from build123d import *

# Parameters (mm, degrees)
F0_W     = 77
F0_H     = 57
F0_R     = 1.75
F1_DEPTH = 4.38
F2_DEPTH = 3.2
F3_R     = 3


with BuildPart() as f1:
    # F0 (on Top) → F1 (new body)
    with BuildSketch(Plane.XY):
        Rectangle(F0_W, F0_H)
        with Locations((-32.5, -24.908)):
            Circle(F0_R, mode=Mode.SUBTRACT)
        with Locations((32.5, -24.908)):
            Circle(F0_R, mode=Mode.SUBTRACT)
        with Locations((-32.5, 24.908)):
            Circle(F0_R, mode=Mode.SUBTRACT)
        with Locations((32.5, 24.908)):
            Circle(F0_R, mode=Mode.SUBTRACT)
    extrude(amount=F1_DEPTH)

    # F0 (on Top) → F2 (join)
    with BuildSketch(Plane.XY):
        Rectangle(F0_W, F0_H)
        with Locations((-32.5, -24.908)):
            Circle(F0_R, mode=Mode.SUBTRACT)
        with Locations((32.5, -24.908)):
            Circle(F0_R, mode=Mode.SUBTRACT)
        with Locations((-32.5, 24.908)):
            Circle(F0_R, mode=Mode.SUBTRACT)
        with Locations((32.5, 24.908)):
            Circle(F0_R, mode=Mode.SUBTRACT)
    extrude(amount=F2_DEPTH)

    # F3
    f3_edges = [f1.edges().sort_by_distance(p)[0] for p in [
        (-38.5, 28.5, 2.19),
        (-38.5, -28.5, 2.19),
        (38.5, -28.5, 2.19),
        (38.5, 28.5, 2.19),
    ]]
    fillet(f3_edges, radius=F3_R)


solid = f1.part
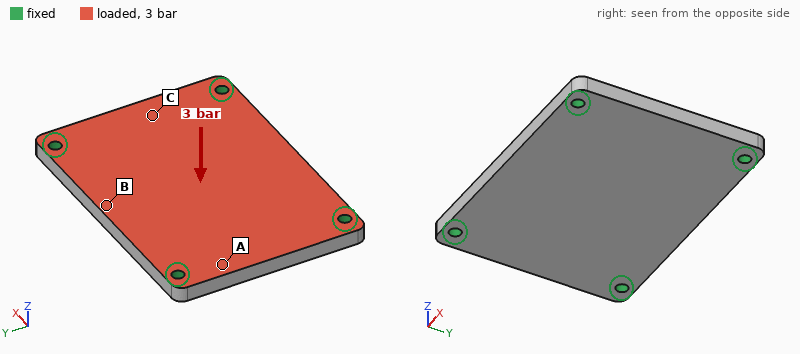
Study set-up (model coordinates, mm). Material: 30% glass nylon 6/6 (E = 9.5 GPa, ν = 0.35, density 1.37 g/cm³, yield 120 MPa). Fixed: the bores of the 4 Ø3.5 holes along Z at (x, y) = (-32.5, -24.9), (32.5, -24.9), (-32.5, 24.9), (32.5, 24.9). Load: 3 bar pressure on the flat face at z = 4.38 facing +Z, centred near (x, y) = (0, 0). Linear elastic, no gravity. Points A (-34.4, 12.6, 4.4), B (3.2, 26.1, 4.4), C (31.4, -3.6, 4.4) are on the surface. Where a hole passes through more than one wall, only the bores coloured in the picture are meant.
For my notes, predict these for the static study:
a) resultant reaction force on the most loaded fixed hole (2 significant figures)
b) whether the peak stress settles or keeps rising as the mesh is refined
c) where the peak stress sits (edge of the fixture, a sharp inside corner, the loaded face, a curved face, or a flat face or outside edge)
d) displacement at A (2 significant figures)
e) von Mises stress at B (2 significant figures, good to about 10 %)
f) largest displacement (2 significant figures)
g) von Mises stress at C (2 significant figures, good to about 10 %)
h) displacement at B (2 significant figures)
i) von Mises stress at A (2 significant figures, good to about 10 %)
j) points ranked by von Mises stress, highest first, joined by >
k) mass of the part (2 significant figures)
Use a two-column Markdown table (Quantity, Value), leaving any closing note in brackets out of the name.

| Quantity | Value |
|---|---|
| resultant reaction force on the most loaded fixed hole | 330 N |
| whether the peak stress settles or keeps rising as the mesh is refined | keeps rising |
| where the peak stress sits | edge of the fixture |
| displacement at A | 0.061 mm |
| von Mises stress at B | 22 MPa |
| largest displacement | 0.39 mm |
| von Mises stress at C | 13 MPa |
| displacement at B | 0.31 mm |
| von Mises stress at A | 7.5 MPa |
| points ranked by von Mises stress, highest first, joined by > | B > C > A |
| mass of the part | 26 g |
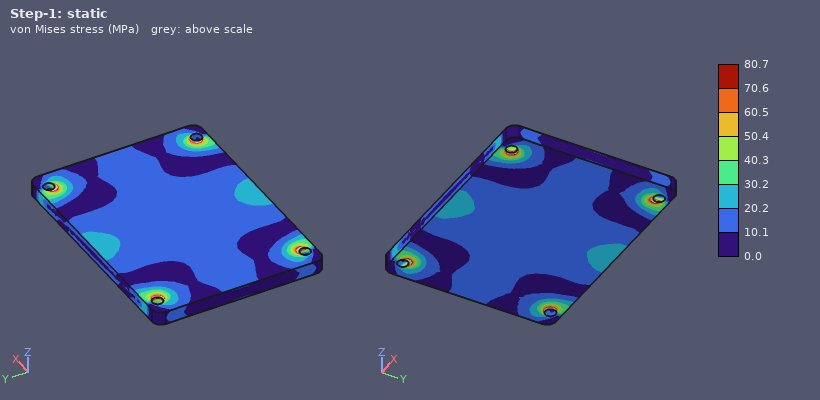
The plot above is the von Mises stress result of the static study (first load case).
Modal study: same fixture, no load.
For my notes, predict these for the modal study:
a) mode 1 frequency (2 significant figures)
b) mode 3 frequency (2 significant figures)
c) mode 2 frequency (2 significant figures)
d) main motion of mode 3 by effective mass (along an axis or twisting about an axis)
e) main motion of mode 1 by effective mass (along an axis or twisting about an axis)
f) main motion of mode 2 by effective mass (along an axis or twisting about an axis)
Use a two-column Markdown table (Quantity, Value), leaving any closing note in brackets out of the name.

| Quantity | Value |
|---|---|
| mode 1 frequency | 2100 Hz |
| mode 3 frequency | 4500 Hz |
| mode 2 frequency | 3400 Hz |
| main motion of mode 3 by effective mass | twisting about Y |
| main motion of mode 1 by effective mass | along Z |
| main motion of mode 2 by effective mass | twisting about X |
